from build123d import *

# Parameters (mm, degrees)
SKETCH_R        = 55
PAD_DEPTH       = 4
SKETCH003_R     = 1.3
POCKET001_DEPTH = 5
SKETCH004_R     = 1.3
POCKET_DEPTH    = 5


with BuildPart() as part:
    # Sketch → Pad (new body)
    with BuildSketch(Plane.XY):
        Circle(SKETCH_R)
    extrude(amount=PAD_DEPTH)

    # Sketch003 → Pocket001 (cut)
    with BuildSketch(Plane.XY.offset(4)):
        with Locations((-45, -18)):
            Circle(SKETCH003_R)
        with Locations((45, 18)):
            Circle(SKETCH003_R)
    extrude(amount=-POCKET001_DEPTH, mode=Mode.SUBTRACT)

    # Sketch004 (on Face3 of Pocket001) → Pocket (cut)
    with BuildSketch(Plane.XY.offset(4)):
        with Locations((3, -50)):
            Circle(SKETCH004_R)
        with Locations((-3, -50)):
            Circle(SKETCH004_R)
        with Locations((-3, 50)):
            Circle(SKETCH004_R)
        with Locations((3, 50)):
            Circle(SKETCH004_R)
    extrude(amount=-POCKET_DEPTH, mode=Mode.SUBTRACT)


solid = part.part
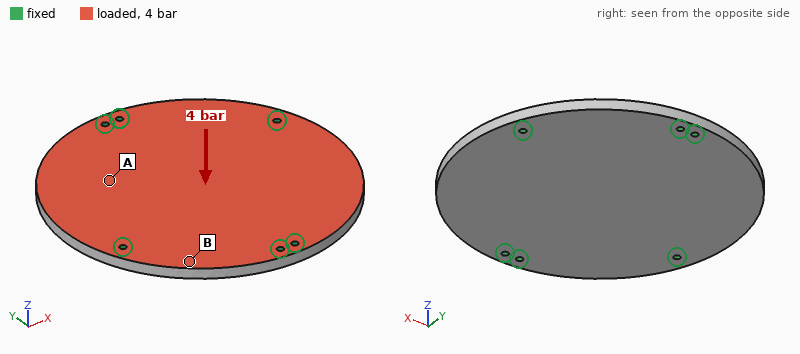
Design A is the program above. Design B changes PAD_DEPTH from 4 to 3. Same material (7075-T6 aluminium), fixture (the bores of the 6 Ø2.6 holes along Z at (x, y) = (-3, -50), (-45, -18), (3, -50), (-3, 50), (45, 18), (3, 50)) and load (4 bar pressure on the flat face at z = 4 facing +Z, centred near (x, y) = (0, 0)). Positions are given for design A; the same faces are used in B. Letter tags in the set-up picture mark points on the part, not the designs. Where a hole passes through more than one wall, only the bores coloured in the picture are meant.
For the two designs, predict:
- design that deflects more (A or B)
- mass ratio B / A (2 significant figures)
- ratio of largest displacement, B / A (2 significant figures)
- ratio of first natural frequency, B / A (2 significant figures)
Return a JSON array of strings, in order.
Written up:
["B", "0.75", "2.3", "0.77"]
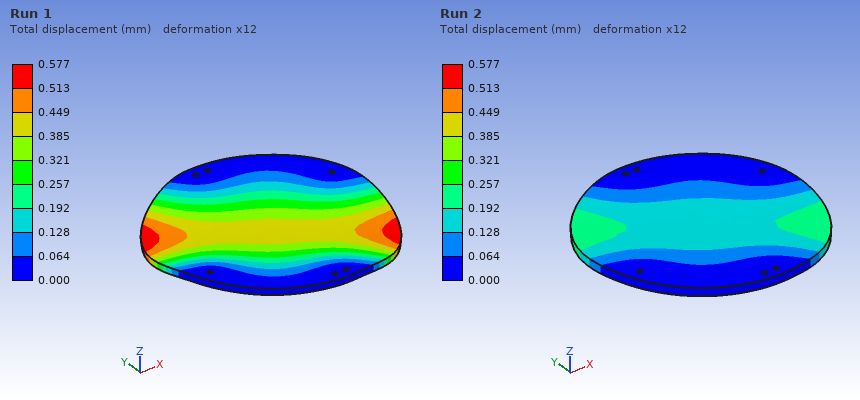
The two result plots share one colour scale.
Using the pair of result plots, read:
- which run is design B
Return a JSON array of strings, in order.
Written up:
["Run 1"]
